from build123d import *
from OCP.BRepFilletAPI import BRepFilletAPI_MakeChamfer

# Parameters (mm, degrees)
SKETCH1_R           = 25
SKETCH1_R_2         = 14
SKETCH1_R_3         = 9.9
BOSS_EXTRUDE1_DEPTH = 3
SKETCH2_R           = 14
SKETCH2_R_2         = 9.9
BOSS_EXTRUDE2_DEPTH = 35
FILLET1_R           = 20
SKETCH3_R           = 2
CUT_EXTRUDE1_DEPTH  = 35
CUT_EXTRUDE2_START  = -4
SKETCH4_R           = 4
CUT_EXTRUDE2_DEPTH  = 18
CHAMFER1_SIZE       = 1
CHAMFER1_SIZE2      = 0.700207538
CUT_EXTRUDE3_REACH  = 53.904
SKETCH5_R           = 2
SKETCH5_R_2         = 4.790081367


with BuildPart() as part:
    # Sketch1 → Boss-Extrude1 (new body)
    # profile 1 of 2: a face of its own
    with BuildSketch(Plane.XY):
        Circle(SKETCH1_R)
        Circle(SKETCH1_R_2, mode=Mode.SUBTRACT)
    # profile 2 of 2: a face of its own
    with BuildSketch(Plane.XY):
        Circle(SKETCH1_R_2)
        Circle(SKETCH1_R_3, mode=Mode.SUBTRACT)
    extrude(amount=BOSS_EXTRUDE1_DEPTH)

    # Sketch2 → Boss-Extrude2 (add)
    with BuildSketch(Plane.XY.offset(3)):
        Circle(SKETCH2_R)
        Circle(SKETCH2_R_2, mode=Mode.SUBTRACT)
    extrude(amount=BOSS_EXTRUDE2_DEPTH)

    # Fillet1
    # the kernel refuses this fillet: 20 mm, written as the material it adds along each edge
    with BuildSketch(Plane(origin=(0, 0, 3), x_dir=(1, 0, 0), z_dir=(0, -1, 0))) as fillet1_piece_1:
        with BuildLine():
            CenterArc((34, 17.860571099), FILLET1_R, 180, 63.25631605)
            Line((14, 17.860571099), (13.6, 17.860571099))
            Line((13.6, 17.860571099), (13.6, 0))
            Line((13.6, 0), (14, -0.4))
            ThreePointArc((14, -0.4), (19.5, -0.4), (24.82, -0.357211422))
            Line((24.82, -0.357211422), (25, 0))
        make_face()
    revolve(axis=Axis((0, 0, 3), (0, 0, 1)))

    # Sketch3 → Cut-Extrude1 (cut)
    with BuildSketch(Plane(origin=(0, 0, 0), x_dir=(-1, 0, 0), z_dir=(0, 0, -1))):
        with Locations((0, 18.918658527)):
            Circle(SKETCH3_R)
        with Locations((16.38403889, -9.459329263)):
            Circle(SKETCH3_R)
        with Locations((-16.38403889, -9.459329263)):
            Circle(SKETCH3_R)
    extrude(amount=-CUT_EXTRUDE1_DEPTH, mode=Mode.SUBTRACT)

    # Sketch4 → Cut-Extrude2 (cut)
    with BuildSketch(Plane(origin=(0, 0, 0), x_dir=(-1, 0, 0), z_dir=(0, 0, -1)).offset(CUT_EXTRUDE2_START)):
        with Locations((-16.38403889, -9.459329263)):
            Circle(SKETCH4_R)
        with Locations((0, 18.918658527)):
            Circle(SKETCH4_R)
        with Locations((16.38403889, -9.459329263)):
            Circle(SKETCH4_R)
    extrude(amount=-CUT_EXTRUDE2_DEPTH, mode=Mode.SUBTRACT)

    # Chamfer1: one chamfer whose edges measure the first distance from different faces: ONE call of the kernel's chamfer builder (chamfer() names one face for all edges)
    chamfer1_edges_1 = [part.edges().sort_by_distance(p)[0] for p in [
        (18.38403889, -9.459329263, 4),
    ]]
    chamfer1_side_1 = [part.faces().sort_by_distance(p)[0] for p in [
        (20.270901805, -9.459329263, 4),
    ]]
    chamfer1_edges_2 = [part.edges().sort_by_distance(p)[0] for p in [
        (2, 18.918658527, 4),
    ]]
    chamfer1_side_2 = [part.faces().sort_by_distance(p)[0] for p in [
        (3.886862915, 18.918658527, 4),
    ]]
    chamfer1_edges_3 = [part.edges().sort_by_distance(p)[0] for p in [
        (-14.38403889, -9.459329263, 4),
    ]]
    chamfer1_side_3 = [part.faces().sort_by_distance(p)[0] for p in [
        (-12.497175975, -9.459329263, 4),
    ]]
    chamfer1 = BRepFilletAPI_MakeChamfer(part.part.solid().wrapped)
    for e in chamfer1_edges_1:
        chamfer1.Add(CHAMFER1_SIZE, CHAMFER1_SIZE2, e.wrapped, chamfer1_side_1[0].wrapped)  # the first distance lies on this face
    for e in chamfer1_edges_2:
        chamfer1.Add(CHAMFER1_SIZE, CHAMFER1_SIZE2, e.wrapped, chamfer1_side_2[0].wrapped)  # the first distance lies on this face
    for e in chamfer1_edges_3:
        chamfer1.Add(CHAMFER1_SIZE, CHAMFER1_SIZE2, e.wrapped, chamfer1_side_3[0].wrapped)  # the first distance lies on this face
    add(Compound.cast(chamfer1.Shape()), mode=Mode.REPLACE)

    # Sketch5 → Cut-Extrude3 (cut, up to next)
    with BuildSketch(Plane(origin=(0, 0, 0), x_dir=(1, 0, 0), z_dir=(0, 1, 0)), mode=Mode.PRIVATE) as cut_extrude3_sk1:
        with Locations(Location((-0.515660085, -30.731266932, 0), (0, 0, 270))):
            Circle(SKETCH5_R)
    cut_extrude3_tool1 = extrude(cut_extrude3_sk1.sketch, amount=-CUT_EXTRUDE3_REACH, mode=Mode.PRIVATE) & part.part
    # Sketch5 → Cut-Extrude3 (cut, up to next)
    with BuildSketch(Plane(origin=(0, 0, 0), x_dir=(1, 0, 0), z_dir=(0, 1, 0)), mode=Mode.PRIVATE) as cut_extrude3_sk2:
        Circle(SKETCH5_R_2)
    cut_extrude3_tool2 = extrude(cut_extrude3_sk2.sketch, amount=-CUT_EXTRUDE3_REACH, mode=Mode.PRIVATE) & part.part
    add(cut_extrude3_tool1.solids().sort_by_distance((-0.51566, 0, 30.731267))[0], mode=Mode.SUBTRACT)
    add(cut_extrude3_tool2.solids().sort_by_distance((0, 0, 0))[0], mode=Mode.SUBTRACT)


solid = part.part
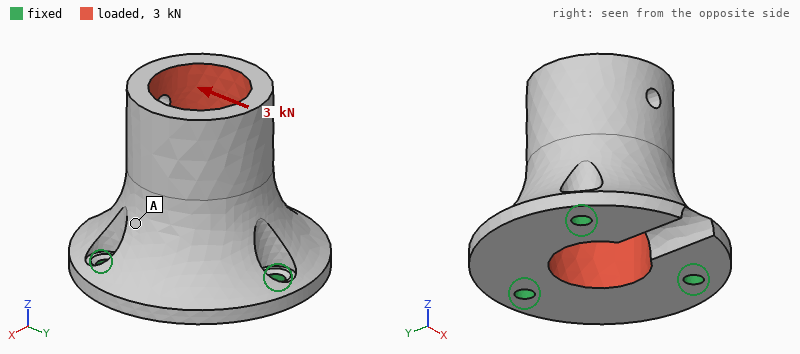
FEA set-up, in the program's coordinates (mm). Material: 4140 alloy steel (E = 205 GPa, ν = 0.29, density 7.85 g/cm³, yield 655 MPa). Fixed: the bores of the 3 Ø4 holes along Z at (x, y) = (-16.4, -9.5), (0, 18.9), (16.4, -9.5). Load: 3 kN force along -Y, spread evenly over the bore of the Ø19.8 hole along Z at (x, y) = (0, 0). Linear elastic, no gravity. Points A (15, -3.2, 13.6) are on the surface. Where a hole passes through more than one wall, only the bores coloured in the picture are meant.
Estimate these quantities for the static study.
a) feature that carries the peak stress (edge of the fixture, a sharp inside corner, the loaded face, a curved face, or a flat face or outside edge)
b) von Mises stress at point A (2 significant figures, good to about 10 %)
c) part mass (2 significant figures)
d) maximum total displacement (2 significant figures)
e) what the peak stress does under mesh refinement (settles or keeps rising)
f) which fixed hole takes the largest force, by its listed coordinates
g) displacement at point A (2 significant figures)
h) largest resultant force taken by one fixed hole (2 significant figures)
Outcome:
edge of the fixture
12 MPa
160 g
11 µm
keeps rising
(0, 18.9)
3.2 µm
2.2 kN
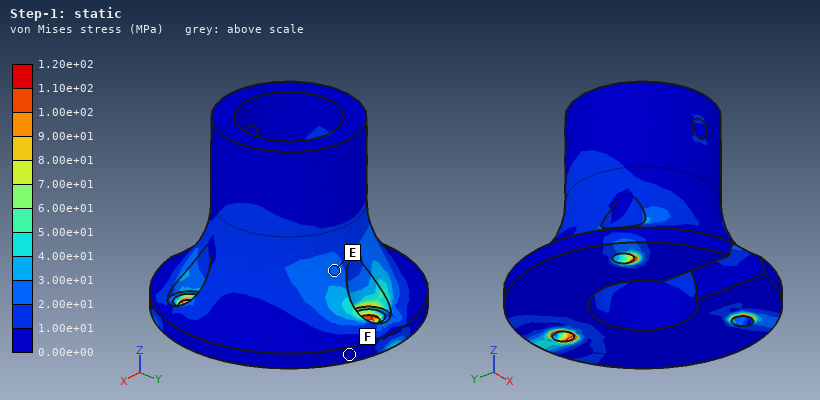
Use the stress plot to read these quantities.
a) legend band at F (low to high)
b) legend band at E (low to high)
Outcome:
0.00e+00 to 1.00e+01 MPa
2.00e+01 to 3.00e+01 MPa
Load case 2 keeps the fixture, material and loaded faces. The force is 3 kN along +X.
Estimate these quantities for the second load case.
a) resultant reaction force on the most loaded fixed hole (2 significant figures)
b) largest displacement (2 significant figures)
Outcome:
2.0 kN
11 µm
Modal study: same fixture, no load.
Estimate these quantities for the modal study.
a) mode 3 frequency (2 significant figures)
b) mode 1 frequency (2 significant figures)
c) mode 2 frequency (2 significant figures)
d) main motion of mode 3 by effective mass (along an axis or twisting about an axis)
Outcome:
17 kHz
9600 Hz
9700 Hz
along Z
